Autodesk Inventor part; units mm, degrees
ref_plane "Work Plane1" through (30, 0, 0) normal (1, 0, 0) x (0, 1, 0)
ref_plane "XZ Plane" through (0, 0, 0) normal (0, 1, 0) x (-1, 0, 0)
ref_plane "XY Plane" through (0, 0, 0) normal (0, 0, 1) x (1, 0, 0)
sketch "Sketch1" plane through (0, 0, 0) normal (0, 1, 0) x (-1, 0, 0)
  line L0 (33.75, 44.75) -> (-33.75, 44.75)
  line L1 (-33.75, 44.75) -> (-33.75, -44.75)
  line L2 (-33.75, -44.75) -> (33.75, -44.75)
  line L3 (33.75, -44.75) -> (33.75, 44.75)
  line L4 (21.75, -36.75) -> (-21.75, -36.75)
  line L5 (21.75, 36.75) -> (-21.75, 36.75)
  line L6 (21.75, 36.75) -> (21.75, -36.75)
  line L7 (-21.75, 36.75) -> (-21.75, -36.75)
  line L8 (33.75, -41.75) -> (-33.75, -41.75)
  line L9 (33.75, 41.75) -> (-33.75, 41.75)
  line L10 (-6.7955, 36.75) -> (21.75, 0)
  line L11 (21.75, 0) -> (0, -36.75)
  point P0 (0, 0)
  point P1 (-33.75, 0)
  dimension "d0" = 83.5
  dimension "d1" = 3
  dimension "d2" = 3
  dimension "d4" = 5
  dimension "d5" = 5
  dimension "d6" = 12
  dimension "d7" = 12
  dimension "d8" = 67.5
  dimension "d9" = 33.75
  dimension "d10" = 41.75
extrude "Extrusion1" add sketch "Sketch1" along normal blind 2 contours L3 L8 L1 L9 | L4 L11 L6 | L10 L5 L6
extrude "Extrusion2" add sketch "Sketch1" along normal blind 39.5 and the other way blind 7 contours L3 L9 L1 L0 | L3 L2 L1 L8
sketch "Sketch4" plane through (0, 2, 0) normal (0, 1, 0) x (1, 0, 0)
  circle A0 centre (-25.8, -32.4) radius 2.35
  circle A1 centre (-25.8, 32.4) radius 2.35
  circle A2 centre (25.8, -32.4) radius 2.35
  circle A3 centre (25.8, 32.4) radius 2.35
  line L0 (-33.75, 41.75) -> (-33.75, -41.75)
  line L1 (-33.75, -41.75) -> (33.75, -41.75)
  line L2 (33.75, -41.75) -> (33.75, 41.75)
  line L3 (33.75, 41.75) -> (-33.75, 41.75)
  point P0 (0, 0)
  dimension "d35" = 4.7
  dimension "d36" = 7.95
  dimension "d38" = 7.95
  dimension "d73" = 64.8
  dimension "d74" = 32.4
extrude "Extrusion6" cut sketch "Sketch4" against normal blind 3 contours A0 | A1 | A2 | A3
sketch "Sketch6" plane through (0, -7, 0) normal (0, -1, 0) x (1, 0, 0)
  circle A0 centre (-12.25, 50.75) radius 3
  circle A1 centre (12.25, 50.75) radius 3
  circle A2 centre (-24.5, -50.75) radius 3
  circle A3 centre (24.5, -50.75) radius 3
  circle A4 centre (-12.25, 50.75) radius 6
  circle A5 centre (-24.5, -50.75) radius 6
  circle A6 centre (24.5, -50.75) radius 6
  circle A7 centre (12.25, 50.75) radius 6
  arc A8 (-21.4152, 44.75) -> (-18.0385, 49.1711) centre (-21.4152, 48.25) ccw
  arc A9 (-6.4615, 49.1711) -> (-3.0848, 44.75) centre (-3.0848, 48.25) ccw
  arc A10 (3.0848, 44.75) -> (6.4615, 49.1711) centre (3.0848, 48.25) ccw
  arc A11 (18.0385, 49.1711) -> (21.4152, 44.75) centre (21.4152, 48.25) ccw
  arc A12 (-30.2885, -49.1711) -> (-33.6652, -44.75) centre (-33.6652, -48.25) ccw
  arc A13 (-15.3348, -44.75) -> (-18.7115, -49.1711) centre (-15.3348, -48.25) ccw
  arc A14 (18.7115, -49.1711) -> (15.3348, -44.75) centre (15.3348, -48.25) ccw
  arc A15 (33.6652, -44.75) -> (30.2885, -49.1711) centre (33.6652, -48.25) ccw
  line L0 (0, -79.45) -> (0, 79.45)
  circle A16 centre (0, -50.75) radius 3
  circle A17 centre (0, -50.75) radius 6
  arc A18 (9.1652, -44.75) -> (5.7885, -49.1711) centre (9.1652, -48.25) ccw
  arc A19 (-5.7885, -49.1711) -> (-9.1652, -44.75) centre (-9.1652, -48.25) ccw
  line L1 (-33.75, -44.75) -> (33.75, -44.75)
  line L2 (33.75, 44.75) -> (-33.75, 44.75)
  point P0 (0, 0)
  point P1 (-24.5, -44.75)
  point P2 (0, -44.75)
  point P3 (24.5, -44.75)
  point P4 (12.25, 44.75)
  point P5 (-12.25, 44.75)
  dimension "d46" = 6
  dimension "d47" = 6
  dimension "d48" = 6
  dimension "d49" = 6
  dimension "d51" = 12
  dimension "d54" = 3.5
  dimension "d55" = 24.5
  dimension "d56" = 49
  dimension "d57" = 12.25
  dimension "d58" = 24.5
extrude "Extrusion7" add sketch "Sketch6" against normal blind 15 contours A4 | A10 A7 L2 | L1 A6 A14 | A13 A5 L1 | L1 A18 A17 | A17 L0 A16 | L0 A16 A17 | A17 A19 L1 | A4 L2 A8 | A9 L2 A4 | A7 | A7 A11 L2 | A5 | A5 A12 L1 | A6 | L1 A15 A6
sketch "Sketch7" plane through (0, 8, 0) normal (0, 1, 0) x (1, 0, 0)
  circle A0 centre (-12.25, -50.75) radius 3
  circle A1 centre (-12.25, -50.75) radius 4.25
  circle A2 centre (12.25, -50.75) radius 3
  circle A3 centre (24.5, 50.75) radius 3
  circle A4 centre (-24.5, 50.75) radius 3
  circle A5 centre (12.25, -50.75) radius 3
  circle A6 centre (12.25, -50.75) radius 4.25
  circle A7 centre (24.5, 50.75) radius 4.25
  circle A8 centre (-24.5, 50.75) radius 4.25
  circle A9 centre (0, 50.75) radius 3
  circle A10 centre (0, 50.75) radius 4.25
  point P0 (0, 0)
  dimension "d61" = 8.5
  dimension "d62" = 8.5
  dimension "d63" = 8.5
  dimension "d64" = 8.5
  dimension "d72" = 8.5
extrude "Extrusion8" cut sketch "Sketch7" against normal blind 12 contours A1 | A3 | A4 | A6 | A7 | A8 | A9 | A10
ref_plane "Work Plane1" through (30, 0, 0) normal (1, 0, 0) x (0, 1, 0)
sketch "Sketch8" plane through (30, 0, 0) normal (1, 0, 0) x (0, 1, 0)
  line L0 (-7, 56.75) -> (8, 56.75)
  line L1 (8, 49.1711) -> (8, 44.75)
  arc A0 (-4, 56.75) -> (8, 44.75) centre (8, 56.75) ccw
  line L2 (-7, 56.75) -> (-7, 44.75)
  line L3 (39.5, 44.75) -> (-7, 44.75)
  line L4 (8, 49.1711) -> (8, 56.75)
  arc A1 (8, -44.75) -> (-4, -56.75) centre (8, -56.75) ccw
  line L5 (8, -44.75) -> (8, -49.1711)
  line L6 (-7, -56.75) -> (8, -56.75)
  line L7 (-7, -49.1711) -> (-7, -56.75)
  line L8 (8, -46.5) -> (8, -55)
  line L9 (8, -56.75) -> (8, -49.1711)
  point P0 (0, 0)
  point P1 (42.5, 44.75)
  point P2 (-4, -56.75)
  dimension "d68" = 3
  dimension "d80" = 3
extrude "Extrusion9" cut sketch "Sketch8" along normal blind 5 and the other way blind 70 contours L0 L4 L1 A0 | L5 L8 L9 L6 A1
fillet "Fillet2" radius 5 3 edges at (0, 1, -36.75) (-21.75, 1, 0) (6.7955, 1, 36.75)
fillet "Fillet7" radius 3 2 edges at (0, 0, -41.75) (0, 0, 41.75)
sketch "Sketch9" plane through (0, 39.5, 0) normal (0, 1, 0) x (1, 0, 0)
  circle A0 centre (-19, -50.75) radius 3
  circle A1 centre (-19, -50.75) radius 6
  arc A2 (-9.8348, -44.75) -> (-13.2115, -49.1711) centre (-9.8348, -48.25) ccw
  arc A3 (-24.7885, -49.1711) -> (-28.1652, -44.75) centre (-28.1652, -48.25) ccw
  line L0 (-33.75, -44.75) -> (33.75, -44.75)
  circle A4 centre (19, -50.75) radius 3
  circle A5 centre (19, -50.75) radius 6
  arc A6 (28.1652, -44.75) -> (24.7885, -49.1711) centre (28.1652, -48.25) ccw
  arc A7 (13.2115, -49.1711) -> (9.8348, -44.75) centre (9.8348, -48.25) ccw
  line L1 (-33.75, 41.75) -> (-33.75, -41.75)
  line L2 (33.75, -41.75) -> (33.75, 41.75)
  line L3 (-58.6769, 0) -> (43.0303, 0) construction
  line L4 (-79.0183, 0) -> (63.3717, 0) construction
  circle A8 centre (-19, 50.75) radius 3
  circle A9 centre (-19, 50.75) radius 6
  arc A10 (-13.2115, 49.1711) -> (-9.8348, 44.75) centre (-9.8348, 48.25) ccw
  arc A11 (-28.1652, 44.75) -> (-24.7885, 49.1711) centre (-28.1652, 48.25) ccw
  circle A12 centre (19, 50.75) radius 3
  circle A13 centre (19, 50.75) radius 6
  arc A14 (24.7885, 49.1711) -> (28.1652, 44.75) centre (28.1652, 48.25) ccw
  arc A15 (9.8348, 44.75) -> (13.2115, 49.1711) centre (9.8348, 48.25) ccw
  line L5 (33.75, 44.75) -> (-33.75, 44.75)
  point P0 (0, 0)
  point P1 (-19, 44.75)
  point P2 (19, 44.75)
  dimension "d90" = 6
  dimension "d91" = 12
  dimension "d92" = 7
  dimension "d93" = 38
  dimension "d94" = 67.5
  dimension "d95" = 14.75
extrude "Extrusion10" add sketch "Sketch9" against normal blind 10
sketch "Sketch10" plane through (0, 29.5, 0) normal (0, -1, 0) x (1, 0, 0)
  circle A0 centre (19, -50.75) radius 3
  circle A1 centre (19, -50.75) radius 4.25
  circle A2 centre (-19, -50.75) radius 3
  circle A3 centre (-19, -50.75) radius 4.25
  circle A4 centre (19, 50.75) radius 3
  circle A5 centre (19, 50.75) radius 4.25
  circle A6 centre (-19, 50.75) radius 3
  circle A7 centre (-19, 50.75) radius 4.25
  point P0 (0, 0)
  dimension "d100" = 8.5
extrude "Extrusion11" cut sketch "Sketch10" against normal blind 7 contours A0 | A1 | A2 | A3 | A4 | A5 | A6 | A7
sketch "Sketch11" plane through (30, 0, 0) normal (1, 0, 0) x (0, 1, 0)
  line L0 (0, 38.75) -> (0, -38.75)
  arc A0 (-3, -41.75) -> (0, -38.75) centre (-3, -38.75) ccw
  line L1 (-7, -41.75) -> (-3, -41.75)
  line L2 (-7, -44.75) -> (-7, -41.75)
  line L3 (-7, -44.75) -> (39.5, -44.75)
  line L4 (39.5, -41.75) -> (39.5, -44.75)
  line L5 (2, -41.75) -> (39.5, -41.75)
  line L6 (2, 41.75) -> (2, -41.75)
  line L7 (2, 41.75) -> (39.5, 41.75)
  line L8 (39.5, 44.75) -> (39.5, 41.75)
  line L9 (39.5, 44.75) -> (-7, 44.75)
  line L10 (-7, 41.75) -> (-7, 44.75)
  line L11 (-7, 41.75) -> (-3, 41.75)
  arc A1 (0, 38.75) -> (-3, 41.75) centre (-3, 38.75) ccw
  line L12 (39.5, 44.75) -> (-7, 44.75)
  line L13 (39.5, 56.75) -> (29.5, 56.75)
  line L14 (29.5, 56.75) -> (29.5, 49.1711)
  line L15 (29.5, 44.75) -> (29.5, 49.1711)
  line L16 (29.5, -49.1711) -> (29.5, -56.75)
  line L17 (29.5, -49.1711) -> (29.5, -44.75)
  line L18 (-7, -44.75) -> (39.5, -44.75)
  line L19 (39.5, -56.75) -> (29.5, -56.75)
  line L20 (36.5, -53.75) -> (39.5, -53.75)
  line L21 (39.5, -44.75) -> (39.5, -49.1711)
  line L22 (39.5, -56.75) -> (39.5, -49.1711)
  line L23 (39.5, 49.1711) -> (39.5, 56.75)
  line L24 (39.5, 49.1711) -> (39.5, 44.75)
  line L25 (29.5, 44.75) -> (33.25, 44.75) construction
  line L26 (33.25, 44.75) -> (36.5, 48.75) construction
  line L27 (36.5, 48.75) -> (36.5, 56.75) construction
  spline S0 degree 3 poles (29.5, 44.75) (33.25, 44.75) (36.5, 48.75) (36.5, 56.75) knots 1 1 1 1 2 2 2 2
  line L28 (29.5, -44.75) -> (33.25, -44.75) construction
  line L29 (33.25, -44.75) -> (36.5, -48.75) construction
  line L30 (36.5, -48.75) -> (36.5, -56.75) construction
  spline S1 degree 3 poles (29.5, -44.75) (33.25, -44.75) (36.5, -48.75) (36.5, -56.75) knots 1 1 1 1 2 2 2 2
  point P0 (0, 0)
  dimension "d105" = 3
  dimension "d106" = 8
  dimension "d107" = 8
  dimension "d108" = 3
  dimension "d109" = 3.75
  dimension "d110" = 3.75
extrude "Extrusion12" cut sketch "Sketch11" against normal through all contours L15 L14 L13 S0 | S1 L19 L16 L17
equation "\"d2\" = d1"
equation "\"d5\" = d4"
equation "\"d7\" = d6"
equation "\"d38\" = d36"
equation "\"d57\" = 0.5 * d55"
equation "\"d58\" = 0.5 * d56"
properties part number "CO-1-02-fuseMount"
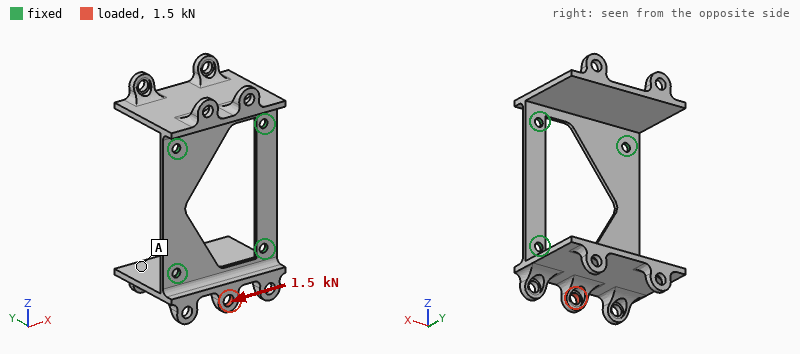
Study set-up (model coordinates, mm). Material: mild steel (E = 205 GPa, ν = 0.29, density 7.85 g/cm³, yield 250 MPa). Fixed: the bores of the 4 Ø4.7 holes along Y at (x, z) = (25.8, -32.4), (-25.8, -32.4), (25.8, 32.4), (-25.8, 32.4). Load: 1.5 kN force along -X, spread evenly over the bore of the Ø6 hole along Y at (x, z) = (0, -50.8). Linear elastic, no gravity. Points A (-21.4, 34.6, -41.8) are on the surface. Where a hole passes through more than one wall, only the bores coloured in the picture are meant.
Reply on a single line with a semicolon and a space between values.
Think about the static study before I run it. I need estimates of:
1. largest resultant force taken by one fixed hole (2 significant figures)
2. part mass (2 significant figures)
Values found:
940 N; 240 g
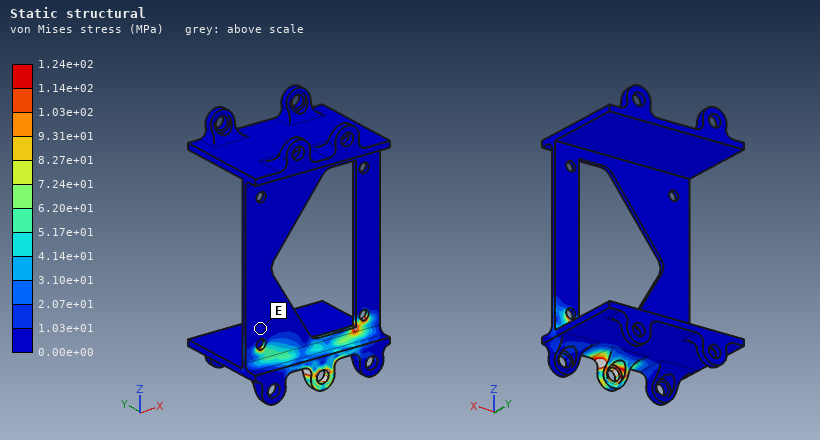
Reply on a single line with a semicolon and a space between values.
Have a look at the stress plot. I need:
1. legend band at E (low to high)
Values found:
0.00e+00 to 1.03e+01 MPa
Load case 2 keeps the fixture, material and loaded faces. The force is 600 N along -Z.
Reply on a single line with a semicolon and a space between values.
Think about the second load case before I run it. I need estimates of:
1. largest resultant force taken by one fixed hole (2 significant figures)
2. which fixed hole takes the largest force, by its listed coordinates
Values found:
430 N; (-25.8, -32.4)
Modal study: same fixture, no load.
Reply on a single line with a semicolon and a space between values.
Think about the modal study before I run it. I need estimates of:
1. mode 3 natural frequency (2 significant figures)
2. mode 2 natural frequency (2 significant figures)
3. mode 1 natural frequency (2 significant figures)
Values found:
2100 Hz; 600 Hz; 590 Hz
